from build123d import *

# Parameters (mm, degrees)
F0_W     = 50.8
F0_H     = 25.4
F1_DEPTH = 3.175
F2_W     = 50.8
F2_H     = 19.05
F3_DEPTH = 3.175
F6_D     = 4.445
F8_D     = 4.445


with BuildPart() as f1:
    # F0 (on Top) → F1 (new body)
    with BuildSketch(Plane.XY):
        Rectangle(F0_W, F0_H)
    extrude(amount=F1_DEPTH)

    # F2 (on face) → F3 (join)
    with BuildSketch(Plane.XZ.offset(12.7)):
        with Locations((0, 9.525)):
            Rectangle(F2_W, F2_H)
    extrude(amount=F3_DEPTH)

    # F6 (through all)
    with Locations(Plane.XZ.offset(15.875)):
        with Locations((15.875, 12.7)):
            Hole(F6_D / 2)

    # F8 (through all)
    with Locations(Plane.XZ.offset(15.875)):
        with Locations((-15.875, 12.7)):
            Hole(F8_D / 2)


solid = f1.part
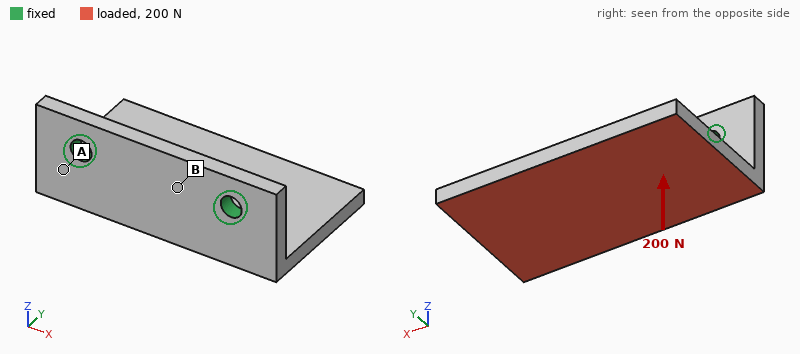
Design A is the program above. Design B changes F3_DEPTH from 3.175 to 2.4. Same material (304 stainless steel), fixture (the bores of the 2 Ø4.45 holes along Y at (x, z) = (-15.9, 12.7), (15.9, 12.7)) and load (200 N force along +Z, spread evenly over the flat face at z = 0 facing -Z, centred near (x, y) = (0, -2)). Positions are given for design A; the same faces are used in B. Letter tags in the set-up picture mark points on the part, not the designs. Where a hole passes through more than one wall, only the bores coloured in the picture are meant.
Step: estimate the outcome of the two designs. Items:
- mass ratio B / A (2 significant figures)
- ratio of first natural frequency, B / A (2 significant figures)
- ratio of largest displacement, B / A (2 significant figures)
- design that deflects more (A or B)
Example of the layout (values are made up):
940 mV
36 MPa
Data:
0.90
0.75
1.8
B
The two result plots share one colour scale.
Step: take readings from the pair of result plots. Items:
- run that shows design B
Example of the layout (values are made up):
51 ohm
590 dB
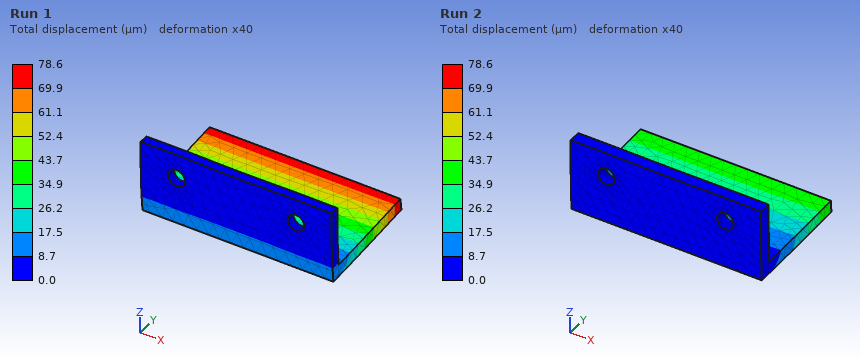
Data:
Run 1
